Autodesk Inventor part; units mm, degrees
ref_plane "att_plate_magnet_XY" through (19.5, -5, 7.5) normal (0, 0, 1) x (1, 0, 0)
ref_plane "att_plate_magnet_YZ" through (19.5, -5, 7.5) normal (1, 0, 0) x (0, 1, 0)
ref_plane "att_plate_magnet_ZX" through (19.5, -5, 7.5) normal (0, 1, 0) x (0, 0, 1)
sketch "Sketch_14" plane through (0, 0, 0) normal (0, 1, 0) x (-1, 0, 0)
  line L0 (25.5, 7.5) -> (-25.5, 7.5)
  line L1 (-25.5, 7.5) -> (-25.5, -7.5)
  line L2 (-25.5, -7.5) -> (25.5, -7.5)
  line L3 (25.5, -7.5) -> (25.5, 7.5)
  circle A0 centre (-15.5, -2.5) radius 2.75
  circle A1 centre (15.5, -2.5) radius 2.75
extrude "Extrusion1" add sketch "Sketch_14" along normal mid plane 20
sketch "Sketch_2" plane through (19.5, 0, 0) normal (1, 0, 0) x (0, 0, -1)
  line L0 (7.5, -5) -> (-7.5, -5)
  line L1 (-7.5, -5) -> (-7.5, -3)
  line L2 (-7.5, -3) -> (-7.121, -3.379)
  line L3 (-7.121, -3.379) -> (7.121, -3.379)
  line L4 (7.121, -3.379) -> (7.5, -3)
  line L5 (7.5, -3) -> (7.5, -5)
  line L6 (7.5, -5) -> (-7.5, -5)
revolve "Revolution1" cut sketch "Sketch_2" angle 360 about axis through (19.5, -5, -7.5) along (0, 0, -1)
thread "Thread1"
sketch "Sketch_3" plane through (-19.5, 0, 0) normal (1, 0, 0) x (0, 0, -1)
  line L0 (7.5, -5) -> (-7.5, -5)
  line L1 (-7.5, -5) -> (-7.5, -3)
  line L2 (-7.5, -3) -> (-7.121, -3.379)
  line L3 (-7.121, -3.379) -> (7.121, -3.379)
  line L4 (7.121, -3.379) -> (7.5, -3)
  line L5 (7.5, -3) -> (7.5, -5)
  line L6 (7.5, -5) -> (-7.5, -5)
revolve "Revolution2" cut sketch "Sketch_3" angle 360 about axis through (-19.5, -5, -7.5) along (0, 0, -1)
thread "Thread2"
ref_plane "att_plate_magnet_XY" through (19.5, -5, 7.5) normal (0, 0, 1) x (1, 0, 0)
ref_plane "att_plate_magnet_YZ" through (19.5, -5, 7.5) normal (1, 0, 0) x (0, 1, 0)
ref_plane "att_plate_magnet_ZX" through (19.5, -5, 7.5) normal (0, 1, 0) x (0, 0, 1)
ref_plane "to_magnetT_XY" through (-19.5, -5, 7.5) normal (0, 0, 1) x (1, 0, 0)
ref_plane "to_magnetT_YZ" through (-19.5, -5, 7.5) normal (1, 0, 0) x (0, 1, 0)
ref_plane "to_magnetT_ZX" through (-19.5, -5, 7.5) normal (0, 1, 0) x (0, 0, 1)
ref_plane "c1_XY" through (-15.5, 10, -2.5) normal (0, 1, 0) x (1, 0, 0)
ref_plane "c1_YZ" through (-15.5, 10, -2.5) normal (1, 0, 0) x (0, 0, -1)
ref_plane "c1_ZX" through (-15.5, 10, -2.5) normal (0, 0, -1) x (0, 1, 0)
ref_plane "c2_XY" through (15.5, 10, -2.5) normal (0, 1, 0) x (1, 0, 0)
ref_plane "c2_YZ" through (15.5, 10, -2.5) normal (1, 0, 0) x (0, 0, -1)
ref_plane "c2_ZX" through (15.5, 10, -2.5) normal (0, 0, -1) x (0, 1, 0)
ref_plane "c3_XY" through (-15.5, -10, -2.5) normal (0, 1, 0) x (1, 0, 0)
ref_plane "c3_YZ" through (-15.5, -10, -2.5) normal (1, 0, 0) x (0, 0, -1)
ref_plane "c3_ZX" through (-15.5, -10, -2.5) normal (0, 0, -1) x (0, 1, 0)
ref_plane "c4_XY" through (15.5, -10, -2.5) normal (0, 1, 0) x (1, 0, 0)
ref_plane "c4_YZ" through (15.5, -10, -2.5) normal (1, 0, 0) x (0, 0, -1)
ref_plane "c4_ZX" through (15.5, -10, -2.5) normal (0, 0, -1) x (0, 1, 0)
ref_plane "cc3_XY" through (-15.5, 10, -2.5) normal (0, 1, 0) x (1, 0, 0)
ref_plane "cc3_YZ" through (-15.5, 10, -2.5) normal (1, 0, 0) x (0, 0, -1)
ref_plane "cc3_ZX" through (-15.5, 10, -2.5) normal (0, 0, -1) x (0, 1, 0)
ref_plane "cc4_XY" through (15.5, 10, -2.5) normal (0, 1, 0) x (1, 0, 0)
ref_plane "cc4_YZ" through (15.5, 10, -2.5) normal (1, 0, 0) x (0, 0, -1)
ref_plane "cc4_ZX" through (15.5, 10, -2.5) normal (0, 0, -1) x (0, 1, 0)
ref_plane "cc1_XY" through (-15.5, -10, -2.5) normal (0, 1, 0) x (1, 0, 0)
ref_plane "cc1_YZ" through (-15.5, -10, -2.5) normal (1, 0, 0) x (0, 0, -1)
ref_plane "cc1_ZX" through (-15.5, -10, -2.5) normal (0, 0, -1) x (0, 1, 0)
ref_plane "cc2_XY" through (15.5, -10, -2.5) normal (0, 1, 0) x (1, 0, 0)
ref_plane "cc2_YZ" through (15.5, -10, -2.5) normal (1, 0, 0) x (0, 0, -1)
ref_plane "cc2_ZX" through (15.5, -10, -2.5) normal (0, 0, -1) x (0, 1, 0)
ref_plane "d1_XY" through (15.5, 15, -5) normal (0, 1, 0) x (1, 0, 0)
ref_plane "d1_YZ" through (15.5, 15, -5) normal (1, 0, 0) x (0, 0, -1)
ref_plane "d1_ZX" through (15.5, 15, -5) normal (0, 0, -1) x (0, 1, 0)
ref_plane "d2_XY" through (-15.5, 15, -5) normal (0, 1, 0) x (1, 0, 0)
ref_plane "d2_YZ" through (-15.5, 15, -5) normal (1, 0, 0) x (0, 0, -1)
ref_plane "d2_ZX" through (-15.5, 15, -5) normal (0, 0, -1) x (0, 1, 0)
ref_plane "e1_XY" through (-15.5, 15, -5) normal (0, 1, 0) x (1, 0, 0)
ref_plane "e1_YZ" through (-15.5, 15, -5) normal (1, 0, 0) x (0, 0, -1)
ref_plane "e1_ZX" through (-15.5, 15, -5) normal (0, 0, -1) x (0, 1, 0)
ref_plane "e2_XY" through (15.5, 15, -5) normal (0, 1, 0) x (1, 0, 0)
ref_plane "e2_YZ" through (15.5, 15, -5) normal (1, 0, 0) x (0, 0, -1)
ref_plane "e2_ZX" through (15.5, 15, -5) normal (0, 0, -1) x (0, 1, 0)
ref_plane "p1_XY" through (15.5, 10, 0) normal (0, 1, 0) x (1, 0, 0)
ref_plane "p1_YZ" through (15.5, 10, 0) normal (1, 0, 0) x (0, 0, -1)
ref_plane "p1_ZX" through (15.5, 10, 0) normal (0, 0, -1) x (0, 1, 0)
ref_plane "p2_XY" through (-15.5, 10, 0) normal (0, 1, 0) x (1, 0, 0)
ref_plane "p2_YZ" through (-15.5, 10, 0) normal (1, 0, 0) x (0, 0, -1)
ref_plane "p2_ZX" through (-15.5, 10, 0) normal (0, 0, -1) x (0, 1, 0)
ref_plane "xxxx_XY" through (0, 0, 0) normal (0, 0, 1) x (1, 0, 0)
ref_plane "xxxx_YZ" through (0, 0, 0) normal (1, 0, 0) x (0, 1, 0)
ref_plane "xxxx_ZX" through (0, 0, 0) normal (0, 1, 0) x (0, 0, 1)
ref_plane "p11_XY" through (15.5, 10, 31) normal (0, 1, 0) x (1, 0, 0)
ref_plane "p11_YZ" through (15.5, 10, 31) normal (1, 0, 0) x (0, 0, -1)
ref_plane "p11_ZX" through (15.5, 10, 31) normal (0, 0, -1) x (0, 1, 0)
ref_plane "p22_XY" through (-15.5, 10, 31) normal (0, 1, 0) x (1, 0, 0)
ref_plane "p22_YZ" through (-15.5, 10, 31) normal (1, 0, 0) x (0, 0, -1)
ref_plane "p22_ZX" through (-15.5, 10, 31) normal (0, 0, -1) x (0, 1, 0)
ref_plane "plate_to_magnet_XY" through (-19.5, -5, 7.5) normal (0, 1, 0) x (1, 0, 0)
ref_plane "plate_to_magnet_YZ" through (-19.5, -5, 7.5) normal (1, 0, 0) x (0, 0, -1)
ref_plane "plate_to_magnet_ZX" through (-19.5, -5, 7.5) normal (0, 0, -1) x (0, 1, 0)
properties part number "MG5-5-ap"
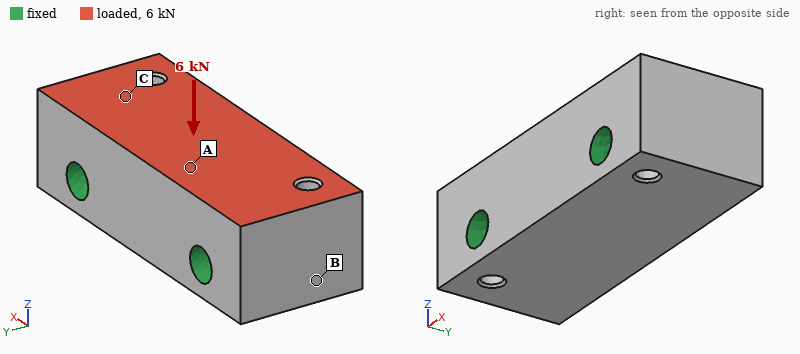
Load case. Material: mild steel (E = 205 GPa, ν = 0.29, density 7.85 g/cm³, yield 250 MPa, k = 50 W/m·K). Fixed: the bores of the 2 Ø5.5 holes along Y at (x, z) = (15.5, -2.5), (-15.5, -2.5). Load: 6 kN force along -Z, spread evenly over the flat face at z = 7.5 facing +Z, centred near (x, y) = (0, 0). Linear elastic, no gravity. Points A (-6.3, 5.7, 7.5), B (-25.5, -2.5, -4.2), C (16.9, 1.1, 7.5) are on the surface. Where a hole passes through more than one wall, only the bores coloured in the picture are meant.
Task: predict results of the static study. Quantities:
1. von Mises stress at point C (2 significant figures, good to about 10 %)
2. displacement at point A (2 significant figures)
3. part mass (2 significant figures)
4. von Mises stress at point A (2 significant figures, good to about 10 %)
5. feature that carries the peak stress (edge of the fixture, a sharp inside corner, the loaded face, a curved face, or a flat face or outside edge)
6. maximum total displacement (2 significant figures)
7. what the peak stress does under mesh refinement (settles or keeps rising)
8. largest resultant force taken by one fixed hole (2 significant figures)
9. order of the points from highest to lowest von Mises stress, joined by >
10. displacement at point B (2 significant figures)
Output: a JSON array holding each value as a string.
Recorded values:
["11 MPa", "0.82 µm", "110 g", "5.8 MPa", "edge of the fixture", "1.0 µm", "keeps rising", "3.0 kN", "C > A > B", "0.35 µm"]
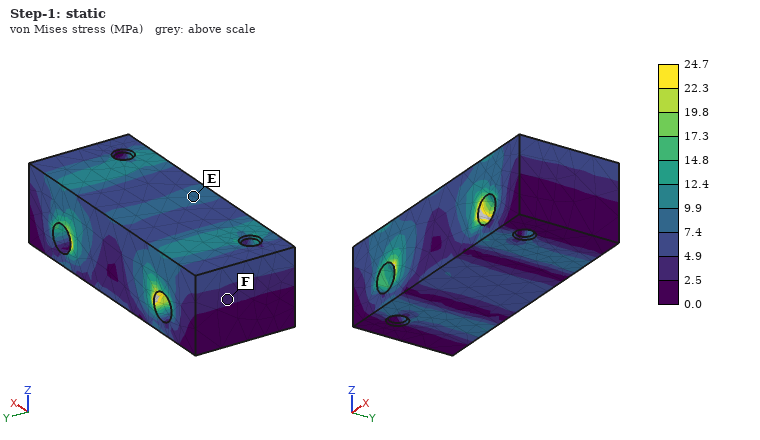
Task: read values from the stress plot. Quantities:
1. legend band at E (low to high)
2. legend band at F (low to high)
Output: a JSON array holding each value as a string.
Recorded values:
["7.4 to 9.9 MPa", "2.5 to 4.9 MPa"]
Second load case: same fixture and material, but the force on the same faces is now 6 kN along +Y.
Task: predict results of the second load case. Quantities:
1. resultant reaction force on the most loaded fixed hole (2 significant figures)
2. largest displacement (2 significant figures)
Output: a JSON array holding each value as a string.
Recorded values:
["3.0 kN", "2.9 µm"]
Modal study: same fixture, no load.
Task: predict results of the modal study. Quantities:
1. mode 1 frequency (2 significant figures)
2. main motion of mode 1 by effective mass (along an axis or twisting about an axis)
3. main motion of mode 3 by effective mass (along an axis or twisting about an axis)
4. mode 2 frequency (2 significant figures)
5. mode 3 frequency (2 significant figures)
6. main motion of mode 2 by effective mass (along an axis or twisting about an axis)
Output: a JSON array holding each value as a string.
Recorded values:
["39 kHz", "along Z", "along X", "43 kHz", "50 kHz", "along Y"]
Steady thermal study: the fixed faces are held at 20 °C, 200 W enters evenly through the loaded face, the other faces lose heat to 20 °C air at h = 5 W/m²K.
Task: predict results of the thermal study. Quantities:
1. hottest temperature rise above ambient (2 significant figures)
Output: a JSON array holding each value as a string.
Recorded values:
["58 K"]
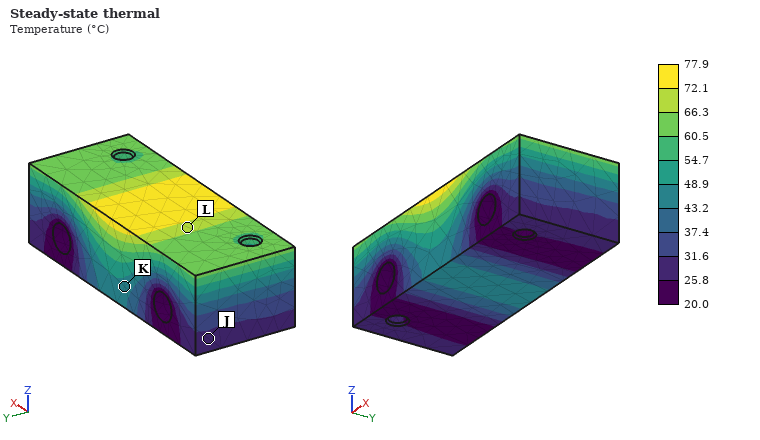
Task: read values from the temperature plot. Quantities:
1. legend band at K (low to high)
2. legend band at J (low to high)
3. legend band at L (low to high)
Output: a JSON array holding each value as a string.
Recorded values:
["43.2 to 48.9 °C", "25.8 to 31.6 °C", "66.3 to 72.1 °C"]
